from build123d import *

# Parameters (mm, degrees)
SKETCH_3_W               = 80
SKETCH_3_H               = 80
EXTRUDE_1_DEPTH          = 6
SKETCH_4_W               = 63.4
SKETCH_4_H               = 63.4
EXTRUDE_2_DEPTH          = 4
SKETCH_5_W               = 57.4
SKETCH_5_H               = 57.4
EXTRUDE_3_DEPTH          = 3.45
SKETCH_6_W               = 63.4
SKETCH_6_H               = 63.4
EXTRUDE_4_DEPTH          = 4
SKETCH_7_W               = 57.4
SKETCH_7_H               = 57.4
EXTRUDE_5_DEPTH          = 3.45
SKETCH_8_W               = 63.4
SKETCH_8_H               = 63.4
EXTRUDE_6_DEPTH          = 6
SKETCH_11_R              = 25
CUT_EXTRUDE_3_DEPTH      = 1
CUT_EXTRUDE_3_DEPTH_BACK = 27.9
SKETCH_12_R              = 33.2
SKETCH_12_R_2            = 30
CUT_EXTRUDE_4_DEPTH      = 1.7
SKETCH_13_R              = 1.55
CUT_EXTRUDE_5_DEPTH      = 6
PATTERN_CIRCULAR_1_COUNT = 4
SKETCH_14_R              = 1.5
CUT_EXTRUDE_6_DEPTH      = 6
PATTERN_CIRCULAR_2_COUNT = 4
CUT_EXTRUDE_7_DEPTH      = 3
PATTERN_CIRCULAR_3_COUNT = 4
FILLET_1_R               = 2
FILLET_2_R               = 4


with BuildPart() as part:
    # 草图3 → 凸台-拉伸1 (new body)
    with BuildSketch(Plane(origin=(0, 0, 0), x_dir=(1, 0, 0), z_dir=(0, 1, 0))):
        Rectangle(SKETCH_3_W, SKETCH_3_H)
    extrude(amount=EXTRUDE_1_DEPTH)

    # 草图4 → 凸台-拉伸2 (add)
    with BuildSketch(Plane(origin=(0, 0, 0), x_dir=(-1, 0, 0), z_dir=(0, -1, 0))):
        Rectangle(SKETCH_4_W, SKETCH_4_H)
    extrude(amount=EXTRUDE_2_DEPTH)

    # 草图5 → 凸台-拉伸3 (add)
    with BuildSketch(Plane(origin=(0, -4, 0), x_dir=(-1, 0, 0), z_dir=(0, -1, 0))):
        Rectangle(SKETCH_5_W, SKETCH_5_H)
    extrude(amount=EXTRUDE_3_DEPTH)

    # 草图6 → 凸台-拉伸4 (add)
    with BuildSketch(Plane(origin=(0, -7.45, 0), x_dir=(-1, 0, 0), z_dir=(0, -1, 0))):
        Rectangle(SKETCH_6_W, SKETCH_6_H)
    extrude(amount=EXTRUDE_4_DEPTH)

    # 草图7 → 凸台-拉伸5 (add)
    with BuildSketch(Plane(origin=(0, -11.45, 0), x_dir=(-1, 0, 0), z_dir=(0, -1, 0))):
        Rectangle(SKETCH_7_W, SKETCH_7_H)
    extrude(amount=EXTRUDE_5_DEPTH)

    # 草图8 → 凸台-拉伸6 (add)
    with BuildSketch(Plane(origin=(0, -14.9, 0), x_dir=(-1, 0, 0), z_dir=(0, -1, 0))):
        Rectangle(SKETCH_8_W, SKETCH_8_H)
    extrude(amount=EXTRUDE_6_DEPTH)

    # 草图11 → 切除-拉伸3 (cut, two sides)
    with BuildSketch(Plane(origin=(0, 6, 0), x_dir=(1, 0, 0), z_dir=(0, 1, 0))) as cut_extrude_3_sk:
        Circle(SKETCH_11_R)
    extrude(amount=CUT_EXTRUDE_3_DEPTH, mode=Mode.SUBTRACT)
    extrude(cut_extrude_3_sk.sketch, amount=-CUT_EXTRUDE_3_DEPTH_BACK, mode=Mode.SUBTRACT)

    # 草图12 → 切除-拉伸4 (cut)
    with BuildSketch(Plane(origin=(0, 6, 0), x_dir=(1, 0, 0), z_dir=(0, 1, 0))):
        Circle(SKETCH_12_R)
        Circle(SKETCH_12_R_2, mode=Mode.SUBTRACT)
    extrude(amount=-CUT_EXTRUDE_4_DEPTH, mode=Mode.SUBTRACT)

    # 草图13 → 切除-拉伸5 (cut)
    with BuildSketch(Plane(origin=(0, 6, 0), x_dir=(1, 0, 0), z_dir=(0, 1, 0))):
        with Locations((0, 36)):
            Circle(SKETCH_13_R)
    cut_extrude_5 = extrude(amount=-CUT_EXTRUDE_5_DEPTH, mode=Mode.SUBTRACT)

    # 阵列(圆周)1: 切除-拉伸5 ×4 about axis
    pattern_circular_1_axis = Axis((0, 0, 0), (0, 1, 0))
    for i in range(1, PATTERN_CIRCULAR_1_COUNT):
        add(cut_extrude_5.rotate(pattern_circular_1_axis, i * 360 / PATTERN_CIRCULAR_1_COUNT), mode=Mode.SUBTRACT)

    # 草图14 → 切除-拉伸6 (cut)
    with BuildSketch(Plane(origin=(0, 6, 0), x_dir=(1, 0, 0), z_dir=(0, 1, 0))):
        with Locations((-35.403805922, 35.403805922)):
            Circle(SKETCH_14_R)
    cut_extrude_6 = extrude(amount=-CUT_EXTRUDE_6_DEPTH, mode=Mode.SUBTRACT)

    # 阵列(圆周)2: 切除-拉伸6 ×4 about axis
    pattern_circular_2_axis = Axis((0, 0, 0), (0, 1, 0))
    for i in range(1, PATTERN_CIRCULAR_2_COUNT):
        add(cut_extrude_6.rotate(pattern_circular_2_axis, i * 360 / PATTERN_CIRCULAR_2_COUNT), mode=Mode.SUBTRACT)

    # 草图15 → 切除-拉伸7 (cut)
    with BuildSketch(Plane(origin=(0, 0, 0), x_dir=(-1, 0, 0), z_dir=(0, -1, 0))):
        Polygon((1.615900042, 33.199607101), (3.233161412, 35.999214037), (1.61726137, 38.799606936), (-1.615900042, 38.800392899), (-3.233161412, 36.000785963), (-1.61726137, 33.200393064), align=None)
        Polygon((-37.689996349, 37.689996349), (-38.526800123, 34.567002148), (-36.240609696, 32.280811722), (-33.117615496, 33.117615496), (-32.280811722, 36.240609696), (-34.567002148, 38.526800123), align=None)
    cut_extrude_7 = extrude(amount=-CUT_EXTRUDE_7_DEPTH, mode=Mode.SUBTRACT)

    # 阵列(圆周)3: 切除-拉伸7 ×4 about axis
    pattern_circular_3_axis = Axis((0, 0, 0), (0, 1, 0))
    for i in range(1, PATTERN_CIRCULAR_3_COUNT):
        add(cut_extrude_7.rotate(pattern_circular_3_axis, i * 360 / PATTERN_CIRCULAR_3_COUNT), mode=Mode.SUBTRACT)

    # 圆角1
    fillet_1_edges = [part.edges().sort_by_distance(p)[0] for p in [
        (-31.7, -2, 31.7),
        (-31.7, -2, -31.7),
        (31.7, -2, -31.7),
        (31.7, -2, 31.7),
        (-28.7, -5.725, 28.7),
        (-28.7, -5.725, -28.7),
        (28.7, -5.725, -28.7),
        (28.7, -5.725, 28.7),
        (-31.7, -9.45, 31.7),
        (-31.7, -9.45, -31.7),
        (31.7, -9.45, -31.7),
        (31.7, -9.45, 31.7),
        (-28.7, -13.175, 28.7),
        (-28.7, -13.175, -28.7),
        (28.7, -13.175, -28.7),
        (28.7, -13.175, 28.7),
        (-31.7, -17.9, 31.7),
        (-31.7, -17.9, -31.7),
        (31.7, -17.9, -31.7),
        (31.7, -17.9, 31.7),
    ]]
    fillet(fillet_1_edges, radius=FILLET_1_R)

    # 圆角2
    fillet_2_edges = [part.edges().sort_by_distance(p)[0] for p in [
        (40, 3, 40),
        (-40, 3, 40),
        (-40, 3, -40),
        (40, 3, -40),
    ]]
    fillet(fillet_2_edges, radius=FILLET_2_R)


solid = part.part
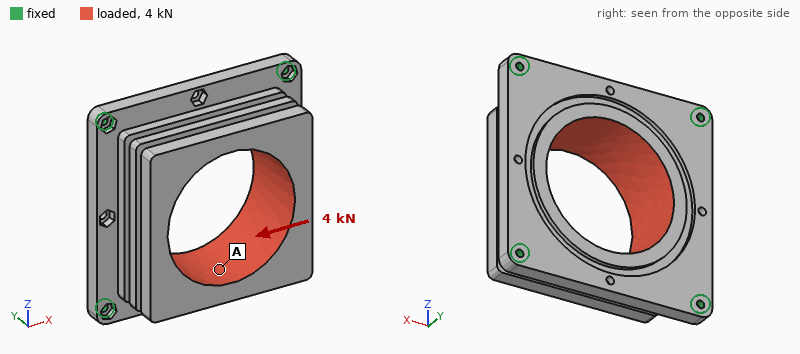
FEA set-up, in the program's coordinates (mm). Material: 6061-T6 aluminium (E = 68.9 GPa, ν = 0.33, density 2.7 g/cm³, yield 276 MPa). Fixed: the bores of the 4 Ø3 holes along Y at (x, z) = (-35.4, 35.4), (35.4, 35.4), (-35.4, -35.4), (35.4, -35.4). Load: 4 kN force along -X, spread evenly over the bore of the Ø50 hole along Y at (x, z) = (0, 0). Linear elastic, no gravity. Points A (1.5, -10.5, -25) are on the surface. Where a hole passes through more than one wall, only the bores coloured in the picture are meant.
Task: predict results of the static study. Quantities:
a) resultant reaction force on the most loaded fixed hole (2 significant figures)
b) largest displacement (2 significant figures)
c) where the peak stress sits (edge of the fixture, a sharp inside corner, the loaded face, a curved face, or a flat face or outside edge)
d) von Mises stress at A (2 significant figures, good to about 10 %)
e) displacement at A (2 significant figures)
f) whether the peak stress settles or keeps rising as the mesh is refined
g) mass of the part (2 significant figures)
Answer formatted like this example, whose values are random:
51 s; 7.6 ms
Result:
1.1 kN; 14 µm; edge of the fixture; 7.0 MPa; 7.1 µm; keeps rising; 170 g
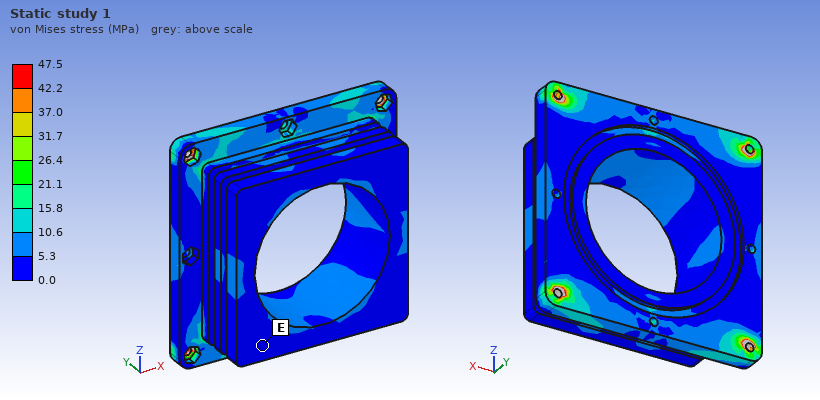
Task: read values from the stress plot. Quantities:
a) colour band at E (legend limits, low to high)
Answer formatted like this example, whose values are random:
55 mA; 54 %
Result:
0.0 to 5.3 MPa
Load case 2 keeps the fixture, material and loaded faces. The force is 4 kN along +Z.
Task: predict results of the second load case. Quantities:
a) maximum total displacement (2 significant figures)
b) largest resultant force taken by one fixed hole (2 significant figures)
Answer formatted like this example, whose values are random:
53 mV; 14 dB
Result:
14 µm; 1.1 kN
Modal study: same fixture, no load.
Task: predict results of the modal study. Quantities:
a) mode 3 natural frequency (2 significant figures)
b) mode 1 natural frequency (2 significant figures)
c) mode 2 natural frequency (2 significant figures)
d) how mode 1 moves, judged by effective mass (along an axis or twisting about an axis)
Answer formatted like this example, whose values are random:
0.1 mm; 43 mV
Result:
6700 Hz; 5300 Hz; 6700 Hz; along Y
